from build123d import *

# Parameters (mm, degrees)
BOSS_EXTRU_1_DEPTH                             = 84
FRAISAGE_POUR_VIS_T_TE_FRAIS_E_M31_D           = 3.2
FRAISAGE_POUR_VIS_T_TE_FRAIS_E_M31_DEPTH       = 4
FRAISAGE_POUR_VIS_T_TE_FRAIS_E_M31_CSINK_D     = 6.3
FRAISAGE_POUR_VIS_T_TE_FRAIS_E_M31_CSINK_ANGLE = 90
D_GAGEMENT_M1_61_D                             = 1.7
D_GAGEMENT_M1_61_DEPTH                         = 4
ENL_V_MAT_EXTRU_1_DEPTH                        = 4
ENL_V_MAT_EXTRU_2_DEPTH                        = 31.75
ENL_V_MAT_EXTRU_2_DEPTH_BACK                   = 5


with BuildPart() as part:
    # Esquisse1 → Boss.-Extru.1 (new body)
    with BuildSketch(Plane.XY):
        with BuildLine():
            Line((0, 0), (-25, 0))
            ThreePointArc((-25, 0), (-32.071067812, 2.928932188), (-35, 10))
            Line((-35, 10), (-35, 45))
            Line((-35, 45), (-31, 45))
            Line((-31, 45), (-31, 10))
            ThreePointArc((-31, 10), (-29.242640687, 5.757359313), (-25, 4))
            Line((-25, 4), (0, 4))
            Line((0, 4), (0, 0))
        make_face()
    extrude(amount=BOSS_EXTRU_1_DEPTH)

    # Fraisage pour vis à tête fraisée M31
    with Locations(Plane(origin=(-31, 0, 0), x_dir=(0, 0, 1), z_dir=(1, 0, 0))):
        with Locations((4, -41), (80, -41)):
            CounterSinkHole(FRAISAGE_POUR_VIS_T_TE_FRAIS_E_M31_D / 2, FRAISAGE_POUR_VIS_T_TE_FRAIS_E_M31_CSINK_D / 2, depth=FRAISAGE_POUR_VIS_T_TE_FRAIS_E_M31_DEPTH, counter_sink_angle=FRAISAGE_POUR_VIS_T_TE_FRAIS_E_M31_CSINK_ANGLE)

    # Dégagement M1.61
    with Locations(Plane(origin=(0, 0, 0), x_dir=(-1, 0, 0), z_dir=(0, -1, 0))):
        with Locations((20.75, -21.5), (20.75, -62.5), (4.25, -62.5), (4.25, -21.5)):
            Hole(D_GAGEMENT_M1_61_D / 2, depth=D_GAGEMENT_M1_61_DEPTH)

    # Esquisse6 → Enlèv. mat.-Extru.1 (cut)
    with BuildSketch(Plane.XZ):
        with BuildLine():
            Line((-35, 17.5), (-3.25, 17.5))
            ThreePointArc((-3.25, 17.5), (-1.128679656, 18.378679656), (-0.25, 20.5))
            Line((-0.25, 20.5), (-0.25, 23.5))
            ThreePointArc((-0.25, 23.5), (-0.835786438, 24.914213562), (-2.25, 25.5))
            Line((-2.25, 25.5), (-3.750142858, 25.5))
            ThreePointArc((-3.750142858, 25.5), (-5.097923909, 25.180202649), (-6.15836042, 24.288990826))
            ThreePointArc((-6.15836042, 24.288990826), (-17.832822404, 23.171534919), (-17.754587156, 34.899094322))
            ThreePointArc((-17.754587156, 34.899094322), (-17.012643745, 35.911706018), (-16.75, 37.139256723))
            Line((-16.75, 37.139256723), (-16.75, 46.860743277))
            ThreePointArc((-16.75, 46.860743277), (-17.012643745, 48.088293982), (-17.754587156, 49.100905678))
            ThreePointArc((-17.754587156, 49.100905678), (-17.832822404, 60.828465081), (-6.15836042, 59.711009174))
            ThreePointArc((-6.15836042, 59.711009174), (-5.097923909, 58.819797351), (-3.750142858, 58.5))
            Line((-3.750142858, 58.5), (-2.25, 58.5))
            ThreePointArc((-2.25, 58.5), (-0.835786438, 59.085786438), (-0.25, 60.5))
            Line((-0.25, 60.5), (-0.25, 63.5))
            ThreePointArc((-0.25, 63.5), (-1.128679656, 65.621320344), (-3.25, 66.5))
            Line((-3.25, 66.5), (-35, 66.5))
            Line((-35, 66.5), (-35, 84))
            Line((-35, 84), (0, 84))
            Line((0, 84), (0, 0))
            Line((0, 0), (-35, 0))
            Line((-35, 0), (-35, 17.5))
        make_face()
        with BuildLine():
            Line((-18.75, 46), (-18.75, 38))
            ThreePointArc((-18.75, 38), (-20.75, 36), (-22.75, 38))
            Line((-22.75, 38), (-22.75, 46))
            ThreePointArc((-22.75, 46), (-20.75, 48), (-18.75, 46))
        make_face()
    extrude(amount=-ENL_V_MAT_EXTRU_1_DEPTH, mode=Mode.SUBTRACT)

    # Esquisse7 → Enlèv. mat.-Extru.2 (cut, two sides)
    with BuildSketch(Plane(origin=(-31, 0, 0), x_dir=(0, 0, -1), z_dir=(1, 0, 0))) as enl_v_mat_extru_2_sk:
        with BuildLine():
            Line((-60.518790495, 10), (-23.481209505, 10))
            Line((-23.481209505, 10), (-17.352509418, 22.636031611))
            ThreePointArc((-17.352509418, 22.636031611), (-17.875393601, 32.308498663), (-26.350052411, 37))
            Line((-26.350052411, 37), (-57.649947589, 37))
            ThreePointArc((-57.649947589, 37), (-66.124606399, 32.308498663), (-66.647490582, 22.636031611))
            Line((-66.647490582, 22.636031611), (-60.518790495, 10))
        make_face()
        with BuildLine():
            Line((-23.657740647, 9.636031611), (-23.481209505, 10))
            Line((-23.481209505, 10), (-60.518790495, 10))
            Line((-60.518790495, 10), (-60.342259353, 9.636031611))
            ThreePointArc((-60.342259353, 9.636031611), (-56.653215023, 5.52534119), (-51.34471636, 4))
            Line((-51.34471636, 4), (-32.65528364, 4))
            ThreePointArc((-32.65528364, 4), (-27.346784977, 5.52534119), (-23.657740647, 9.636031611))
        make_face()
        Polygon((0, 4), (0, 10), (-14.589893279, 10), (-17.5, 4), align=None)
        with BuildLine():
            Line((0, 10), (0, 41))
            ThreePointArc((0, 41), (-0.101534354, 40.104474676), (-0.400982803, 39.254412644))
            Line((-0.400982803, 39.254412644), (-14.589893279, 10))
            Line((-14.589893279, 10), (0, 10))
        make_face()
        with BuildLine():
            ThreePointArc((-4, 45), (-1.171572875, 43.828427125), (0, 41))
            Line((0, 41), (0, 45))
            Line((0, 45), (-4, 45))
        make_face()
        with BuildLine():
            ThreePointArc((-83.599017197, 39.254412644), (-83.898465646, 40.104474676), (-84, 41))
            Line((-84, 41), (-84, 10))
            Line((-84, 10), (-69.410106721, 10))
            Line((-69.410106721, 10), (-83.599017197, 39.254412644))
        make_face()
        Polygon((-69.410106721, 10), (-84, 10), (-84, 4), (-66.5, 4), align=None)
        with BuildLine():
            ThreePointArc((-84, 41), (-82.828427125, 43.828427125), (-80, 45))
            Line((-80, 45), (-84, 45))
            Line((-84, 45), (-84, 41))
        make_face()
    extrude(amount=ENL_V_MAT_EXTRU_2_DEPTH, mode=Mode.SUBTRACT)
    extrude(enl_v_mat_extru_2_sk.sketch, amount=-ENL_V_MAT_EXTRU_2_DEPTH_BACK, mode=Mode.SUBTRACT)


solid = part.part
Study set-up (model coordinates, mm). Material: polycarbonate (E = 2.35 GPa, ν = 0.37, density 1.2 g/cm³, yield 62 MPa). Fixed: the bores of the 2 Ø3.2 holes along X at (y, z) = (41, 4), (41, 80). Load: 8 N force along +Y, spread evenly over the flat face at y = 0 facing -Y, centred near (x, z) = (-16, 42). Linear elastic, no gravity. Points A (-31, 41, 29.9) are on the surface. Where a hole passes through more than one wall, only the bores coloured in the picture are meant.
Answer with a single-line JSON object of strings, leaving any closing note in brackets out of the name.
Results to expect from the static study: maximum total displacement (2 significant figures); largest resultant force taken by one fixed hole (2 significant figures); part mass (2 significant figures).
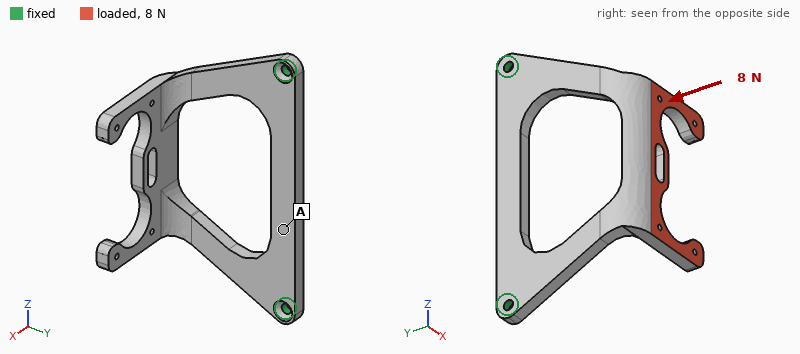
{"maximum total displacement": "1.1 mm", "largest resultant force taken by one fixed hole": "4.5 N", "part mass": "10 g"}
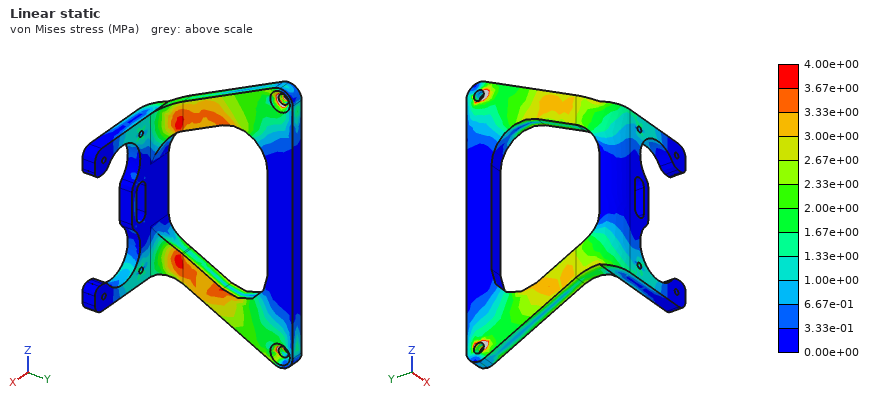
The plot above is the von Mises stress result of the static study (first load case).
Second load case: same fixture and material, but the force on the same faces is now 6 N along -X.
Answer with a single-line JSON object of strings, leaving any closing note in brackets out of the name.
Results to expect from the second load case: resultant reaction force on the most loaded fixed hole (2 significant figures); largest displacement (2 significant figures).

{"resultant reaction force on the most loaded fixed hole": "3.1 N", "largest displacement": "1.0 mm"}
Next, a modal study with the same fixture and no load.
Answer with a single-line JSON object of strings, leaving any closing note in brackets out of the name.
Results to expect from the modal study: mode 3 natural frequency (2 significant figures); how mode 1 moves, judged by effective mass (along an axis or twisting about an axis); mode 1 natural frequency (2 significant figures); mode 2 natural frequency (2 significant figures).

{"mode 3 natural frequency": "700 Hz", "how mode 1 moves, judged by effective mass": "along X", "mode 1 natural frequency": "220 Hz", "mode 2 natural frequency": "490 Hz"}
